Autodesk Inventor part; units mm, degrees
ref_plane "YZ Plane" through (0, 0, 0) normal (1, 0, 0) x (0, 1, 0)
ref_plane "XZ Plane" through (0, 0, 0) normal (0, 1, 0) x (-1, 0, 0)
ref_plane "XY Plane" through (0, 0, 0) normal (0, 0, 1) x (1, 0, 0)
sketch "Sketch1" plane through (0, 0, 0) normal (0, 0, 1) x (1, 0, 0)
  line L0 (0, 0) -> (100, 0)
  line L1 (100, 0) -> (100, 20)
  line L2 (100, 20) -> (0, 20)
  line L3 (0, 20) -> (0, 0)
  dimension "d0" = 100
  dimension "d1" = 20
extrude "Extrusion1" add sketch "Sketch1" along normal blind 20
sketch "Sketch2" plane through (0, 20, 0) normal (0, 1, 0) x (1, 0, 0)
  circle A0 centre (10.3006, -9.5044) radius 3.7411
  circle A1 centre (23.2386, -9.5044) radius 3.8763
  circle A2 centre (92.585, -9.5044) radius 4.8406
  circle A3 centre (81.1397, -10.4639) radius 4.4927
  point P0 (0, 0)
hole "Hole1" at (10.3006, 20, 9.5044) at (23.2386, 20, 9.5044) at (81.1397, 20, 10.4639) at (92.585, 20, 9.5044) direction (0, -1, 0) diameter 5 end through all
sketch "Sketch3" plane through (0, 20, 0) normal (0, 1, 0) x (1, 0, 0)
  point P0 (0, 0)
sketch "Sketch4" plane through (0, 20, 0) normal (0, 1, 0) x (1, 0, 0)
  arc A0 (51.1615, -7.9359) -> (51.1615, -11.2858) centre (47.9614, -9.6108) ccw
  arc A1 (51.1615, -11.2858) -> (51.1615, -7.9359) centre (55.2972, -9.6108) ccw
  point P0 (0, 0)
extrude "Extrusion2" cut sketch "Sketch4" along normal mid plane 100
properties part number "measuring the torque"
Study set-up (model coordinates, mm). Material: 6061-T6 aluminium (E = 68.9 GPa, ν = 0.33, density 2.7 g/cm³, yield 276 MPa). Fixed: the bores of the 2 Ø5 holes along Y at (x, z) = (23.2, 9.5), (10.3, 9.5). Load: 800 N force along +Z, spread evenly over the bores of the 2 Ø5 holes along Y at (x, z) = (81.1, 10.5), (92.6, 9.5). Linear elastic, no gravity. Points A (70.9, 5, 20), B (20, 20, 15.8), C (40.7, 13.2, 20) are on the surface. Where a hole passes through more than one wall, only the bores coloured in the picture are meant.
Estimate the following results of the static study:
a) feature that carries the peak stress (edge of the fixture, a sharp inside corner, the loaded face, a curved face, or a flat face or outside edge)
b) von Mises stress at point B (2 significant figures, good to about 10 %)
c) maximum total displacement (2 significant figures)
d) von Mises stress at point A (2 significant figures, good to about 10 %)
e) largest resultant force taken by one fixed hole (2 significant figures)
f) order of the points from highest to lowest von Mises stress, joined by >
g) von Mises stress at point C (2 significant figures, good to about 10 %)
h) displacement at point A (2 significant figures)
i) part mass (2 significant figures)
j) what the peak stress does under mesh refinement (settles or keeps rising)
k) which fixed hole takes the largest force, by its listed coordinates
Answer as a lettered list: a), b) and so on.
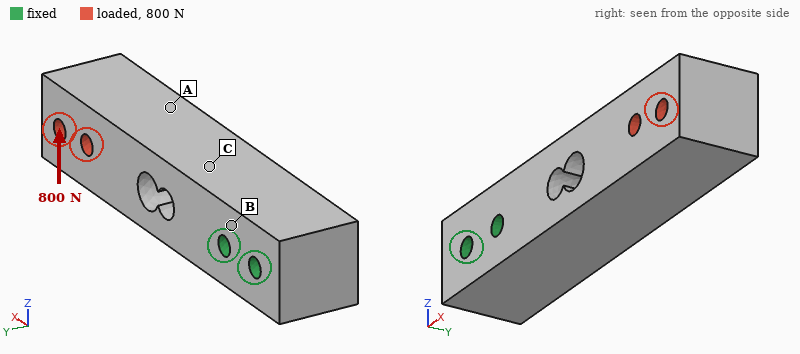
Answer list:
a) edge of the fixture
b) 20 MPa
c) 0.15 mm
d) 9.2 MPa
e) 3.0 kN
f) C > B > A
g) 34 MPa
h) 0.082 mm
i) 98 g
j) keeps rising
k) (23.2, 9.5)
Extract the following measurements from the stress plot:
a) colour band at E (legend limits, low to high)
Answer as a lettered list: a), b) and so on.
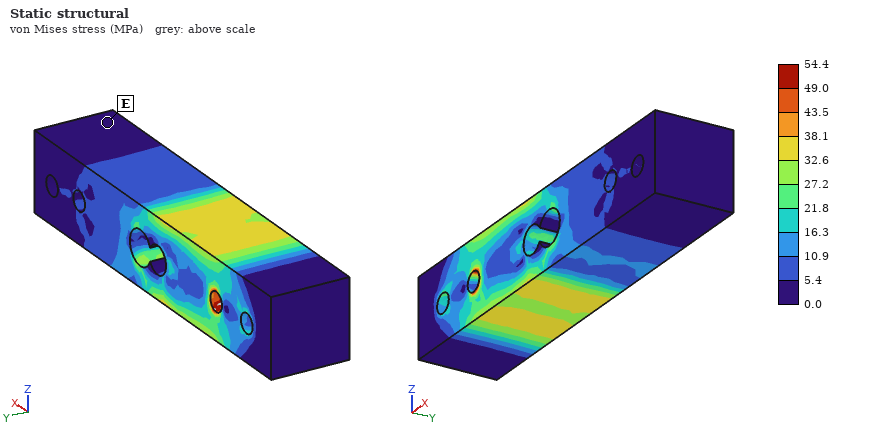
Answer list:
a) 0.0 to 5.4 MPa
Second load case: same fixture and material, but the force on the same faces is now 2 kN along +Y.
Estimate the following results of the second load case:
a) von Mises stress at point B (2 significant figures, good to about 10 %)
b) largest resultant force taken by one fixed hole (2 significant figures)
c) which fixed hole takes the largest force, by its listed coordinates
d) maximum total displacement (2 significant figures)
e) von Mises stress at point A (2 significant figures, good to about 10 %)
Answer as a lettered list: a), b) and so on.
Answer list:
a) 38 MPa
b) 3.2 kN
c) (23.2, 9.5)
d) 0.33 mm
e) 20 MPa
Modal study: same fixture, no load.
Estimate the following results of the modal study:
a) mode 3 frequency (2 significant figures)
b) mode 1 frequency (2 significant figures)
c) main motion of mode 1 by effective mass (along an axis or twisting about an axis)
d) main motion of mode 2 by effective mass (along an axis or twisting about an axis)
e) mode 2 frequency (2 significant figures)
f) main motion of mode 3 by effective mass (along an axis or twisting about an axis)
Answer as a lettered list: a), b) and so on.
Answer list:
a) 8100 Hz
b) 2300 Hz
c) along Z
d) along Y
e) 2500 Hz
f) twisting about X
